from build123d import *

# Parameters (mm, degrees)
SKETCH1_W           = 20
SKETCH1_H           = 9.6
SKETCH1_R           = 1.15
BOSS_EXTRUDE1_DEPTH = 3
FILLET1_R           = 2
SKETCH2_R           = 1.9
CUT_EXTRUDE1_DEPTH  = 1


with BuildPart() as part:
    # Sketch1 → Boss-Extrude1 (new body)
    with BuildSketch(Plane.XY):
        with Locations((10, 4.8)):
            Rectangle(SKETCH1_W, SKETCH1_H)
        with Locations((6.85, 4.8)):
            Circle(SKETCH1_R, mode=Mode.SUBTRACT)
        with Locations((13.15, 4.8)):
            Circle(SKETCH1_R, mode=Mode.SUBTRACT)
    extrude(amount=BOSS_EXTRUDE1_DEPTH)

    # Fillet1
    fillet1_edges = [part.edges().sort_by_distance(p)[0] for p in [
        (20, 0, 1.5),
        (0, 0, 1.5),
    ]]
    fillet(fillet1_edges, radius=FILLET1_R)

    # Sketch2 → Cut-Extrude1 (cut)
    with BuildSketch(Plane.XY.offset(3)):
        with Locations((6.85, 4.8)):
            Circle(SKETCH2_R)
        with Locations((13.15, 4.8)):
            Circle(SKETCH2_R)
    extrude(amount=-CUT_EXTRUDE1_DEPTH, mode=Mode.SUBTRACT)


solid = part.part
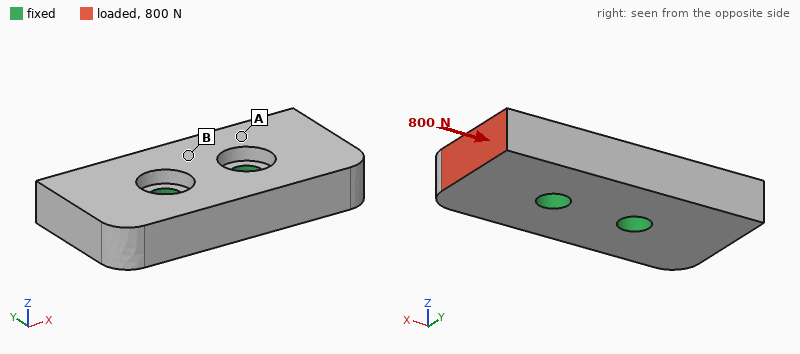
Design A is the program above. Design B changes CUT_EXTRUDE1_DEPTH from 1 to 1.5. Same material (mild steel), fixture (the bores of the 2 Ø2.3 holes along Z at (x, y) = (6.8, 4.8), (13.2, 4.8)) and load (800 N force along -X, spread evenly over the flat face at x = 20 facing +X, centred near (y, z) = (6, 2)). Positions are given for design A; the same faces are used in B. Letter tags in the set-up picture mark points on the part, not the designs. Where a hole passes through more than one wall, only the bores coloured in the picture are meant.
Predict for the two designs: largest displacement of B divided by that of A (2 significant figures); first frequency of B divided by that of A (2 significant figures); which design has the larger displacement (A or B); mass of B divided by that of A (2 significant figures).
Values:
1.3
0.89
B
0.99
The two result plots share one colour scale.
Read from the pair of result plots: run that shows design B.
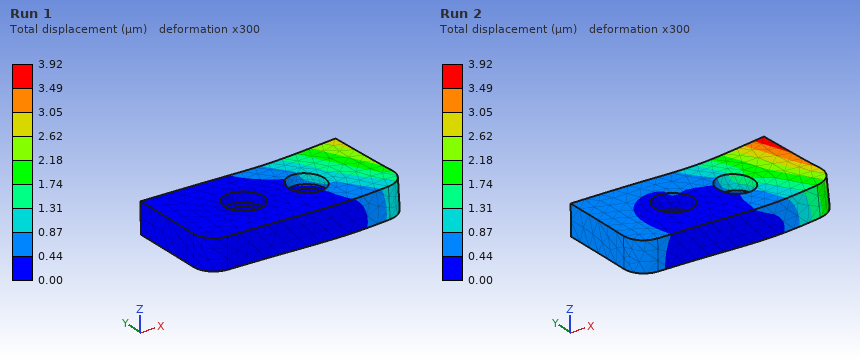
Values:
Run 2
